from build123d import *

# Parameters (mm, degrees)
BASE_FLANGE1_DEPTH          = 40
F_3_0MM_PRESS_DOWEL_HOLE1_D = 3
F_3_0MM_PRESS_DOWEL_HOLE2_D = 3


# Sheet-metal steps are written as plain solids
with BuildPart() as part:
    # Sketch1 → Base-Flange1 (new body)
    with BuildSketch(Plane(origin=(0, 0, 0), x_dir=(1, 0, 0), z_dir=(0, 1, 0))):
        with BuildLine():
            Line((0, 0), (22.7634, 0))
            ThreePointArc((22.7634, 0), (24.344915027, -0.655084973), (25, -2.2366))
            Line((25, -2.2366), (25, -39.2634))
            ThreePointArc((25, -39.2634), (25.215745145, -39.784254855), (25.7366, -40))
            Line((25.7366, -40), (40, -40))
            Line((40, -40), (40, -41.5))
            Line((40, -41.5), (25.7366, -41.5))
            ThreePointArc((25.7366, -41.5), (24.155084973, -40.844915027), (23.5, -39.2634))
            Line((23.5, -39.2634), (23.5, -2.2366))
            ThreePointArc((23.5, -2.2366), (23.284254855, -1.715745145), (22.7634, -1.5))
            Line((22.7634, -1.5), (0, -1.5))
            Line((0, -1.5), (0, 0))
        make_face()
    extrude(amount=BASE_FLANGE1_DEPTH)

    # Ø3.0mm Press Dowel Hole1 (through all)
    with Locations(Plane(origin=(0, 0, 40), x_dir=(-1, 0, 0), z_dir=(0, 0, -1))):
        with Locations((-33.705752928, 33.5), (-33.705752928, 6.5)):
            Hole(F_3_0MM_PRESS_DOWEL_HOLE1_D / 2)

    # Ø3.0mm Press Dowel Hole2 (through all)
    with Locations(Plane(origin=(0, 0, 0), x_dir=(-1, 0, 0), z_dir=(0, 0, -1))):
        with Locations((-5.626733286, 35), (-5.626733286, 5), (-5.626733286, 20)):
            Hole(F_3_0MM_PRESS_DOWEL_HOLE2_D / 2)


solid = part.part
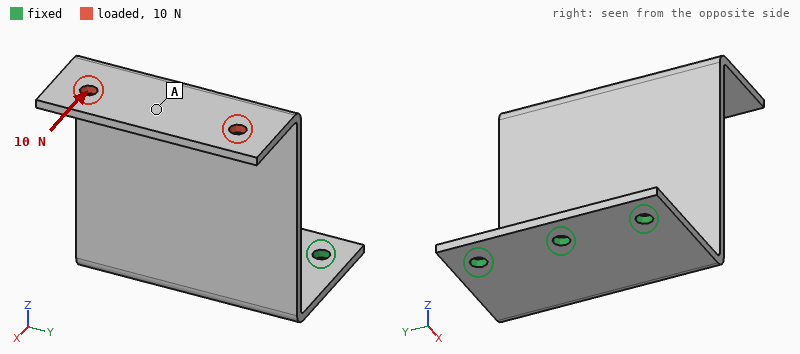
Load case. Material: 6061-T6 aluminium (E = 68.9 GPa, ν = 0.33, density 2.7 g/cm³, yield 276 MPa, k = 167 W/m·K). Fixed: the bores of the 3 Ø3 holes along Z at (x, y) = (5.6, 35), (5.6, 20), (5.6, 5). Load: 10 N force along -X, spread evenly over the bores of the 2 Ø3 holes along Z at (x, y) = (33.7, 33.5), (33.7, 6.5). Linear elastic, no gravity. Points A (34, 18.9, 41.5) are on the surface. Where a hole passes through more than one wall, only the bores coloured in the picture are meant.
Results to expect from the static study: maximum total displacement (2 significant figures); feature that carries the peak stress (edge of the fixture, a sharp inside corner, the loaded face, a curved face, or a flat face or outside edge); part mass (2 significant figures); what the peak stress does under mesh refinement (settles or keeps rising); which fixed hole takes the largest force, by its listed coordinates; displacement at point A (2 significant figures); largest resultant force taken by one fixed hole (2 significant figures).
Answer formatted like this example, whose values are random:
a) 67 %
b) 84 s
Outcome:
a) 0.70 mm
b) edge of the fixture
c) 13 g
d) keeps rising
e) (5.6, 20)
f) 0.65 mm
g) 5.9 N
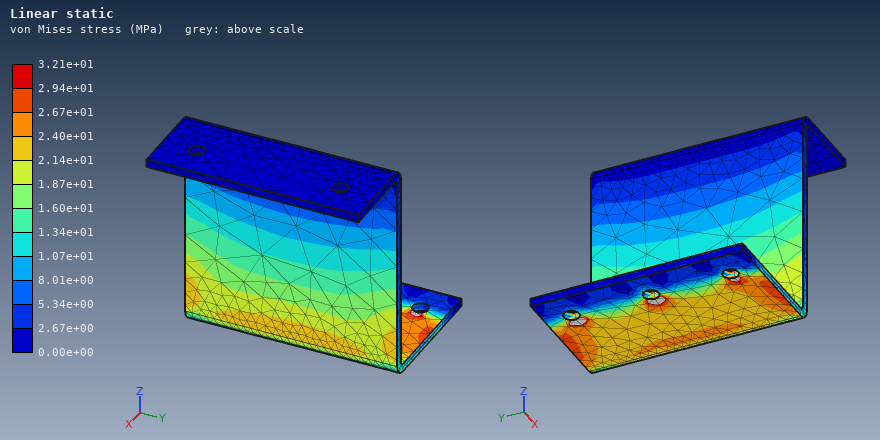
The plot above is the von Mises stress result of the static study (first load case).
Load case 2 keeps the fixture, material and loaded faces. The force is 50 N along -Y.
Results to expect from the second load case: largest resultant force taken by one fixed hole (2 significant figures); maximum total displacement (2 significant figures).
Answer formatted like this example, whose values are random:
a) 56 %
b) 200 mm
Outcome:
a) 80 N
b) 0.53 mm
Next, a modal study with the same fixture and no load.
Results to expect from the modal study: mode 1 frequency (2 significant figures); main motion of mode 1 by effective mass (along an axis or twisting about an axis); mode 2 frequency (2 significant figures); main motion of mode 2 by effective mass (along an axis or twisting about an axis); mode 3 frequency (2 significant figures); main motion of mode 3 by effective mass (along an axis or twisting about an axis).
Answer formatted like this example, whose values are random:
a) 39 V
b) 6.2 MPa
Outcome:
a) 300 Hz
b) along X
c) 750 Hz
d) along Y
e) 1100 Hz
f) twisting about Z
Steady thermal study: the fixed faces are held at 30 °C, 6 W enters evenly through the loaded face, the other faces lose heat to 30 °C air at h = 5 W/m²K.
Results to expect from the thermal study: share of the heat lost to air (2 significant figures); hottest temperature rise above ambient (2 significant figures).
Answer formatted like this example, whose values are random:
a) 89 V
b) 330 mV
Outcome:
a) 10 %
b) 40 K
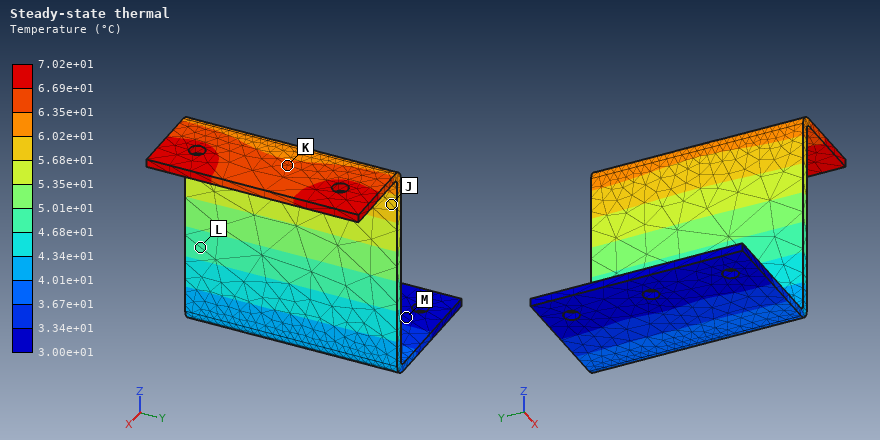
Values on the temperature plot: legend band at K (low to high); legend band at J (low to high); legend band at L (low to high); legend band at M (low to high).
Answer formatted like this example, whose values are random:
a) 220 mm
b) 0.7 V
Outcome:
a) 6.35e+01 to 6.69e+01 °C
b) 5.68e+01 to 6.02e+01 °C
c) 4.68e+01 to 5.01e+01 °C
d) 3.00e+01 to 3.34e+01 °C
